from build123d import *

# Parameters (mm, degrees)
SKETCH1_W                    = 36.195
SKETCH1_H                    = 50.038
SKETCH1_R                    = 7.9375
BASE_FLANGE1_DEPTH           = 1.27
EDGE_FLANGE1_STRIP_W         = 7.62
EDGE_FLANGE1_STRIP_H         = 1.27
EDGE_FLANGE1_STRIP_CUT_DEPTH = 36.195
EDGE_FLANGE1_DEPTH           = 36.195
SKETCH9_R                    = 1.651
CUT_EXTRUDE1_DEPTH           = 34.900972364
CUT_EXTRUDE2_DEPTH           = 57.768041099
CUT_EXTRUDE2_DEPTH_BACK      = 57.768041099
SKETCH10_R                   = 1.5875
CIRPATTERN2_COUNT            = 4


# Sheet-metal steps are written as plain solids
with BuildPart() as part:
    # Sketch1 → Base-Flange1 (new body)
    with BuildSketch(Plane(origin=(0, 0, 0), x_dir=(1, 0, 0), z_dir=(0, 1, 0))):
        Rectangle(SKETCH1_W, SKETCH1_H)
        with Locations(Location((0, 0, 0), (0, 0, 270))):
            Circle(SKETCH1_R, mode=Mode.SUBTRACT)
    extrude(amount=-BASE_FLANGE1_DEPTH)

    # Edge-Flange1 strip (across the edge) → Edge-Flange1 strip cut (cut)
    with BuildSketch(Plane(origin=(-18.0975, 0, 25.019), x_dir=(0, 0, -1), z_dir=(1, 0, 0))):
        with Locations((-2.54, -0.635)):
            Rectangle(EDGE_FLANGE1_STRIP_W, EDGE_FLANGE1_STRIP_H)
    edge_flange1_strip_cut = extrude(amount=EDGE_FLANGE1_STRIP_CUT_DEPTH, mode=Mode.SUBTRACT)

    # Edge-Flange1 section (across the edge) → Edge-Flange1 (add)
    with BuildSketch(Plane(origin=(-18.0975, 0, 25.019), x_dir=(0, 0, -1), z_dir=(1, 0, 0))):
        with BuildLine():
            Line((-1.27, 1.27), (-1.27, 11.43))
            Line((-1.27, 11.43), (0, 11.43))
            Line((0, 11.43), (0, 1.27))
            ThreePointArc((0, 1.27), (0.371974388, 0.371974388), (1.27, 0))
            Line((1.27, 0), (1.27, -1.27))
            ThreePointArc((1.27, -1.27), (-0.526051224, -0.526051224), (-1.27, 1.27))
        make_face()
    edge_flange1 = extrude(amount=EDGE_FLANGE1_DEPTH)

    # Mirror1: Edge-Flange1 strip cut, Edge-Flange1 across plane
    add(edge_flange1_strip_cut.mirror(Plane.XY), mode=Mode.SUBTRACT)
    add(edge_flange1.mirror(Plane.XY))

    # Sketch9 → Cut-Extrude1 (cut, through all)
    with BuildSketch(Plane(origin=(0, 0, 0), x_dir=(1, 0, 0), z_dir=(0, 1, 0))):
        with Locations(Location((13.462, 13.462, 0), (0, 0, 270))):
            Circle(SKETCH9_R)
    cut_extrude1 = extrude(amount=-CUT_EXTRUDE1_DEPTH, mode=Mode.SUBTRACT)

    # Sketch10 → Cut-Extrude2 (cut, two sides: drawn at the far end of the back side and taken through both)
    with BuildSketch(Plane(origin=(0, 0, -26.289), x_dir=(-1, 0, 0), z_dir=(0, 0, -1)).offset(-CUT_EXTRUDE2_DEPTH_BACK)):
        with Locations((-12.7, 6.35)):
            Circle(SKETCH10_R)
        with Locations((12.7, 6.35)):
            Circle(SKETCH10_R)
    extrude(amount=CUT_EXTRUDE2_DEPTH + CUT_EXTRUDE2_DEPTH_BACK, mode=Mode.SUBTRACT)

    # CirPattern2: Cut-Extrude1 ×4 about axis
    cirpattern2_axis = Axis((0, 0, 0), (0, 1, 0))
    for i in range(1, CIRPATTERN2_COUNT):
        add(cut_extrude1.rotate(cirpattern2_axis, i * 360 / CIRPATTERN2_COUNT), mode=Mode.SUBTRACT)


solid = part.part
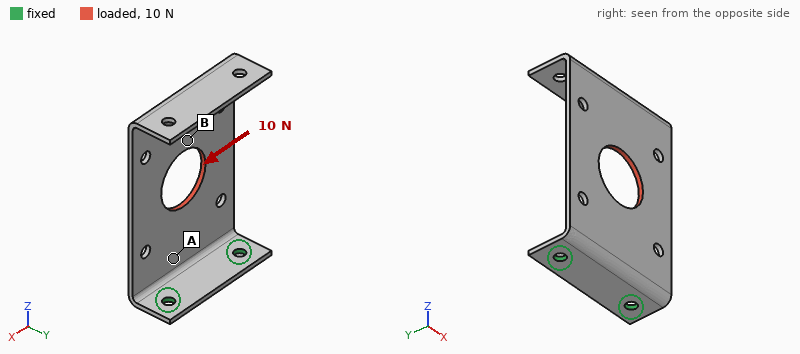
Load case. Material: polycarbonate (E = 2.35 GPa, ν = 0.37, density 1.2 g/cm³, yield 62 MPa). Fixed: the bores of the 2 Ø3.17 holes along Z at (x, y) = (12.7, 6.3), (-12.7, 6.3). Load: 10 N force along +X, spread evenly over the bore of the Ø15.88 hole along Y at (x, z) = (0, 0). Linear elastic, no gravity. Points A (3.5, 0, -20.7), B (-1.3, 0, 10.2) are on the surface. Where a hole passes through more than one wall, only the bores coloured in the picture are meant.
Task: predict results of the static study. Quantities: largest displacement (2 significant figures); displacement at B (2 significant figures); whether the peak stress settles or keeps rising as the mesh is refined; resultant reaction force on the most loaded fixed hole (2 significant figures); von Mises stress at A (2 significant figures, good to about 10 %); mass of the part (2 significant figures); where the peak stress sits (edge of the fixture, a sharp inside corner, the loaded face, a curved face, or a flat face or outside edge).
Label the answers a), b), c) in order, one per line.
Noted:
a) 0.72 mm
b) 0.32 mm
c) keeps rising
d) 11 N
e) 2.6 MPa
f) 3.7 g
g) edge of the fixture
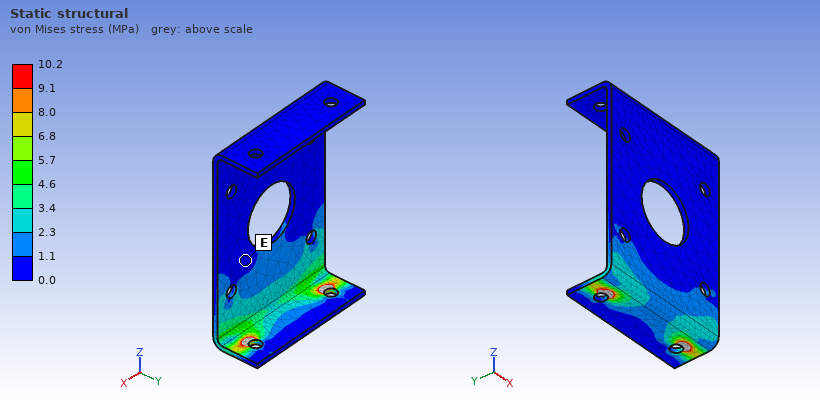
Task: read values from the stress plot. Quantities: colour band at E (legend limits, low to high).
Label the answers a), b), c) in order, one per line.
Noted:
a) 0.0 to 1.1 MPa
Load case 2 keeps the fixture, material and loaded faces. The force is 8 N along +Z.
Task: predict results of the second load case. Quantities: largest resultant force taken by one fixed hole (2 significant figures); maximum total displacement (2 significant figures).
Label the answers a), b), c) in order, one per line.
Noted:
a) 4.0 N
b) 0.63 mm
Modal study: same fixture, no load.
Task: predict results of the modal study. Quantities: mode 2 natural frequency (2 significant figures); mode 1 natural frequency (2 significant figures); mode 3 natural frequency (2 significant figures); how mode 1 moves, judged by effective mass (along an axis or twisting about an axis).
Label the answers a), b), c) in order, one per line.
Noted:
a) 220 Hz
b) 66 Hz
c) 410 Hz
d) along Y
